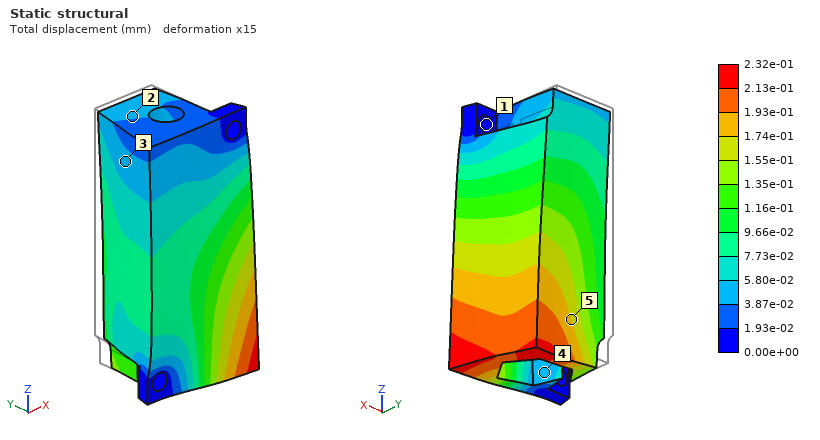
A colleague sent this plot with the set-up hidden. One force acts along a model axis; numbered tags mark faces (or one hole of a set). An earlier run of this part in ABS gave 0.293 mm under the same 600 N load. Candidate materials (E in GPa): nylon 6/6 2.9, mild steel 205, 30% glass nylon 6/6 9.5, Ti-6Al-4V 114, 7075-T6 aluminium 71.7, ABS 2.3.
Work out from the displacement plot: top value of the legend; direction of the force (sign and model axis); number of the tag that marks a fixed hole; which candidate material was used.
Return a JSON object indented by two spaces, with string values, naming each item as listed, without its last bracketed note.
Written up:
{
  "top value of the legend": "2.32e-01 mm",
  "direction of the force": "-Y",
  "number of the tag that marks a fixed hole": "1",
  "which candidate material was used": "nylon 6/6"
}
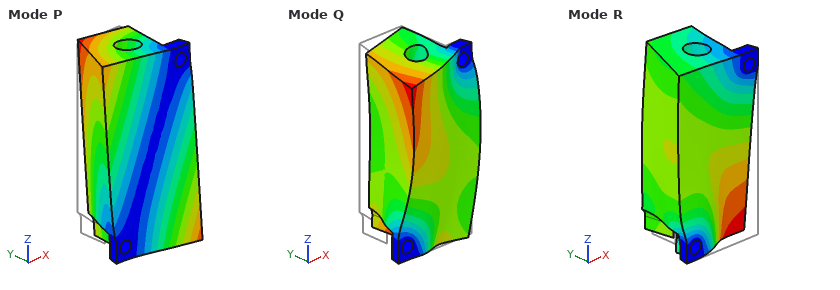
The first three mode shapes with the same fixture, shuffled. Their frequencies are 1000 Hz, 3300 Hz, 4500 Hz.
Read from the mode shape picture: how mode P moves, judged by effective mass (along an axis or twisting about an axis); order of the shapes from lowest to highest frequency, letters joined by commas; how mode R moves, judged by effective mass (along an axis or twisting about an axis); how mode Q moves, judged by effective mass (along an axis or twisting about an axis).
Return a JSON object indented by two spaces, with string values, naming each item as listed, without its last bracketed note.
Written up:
{
  "how mode P moves, judged by effective mass": "along X",
  "order of the shapes from lowest to highest frequency, letters joined by commas": "P, R, Q",
  "how mode R moves, judged by effective mass": "along Y",
  "how mode Q moves, judged by effective mass": "along X"
}
